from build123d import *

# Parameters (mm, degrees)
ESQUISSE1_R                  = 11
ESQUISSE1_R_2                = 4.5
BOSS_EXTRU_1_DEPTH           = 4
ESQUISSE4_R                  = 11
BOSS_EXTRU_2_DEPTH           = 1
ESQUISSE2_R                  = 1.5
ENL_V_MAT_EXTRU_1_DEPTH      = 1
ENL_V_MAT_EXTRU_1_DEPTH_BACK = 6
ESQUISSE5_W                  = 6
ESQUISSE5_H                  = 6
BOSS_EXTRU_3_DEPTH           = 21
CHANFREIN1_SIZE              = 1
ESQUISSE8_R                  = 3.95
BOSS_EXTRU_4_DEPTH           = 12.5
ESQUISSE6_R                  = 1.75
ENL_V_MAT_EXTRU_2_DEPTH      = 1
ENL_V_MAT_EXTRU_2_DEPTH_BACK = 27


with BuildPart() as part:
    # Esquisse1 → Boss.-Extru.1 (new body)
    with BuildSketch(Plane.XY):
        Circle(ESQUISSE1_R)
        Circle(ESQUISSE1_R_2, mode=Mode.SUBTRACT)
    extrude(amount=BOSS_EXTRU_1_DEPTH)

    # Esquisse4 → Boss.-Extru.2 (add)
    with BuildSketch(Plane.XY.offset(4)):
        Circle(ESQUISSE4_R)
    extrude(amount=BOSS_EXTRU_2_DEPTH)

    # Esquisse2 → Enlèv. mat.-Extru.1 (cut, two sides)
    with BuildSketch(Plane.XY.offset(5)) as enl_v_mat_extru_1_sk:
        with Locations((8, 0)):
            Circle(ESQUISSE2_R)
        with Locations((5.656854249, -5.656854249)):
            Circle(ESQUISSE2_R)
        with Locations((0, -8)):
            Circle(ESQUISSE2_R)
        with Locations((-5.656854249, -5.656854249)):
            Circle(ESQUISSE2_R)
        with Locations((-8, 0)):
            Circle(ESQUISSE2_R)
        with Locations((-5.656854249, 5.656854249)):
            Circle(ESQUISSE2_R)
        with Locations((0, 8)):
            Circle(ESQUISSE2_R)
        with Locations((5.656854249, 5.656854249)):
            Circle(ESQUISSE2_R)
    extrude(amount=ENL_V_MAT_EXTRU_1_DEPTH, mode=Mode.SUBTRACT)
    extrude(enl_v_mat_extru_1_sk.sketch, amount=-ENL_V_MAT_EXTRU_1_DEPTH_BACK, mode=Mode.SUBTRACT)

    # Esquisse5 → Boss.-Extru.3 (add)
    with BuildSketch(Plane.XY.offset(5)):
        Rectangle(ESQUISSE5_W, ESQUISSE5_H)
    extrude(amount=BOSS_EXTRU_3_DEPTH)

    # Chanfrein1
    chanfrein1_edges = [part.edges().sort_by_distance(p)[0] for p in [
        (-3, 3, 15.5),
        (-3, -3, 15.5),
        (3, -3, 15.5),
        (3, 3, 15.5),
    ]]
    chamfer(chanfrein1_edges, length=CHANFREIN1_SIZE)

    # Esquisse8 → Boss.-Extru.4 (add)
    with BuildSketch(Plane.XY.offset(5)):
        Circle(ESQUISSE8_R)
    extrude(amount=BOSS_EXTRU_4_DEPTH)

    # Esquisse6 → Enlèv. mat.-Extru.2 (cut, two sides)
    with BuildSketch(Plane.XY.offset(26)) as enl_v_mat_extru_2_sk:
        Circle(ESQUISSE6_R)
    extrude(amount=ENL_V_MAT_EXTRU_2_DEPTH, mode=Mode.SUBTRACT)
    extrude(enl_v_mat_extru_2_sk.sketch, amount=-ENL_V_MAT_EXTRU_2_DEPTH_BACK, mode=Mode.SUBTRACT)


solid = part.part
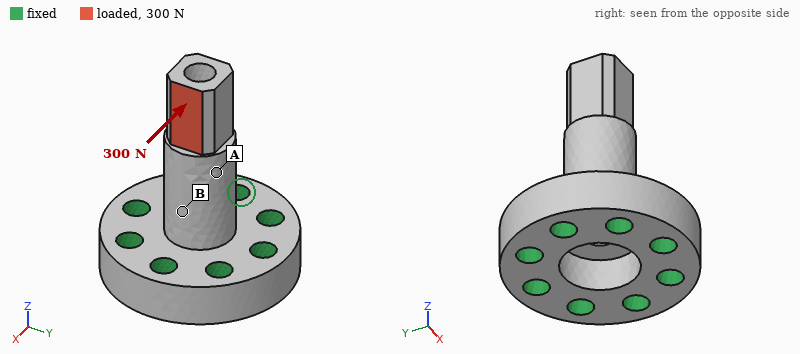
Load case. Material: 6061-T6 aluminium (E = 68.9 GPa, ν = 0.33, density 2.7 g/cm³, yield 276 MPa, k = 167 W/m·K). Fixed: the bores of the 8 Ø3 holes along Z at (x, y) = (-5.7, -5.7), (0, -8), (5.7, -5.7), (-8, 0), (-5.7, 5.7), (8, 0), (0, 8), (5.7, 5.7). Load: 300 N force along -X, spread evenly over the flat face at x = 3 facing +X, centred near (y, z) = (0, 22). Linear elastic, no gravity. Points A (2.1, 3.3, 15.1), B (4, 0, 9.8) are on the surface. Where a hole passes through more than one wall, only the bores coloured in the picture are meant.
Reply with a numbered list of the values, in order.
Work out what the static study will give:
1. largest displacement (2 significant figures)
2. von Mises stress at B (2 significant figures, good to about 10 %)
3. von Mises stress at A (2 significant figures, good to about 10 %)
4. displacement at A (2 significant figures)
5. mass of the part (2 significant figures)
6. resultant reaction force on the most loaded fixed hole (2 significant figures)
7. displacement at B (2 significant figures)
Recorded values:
1. 0.11 mm
2. 76 MPa
3. 26 MPa
4. 0.043 mm
5. 5.5 g
6. 290 N
7. 0.023 mm
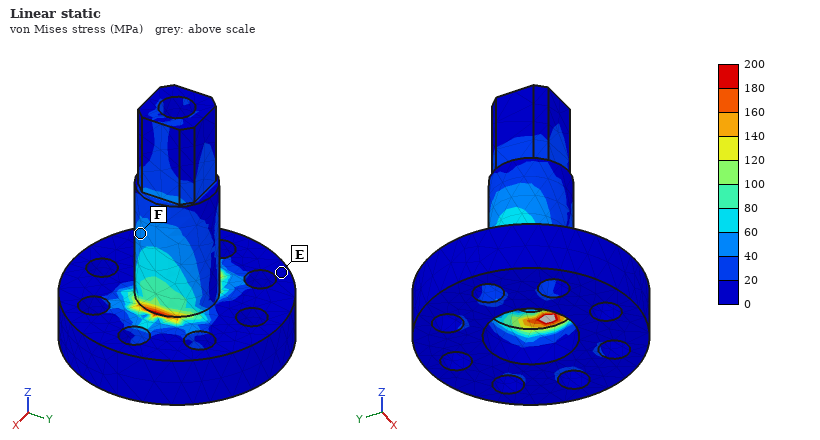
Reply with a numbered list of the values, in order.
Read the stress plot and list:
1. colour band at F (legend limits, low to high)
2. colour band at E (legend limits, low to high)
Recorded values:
1. 40 to 60 MPa
2. 0 to 20 MPa
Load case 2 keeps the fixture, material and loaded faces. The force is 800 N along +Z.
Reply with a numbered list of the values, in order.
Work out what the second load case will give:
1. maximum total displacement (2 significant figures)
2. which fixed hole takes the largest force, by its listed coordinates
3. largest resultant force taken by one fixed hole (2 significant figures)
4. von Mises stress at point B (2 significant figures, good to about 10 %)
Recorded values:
1. 77 µm
2. (8, 0)
3. 250 N
4. 69 MPa
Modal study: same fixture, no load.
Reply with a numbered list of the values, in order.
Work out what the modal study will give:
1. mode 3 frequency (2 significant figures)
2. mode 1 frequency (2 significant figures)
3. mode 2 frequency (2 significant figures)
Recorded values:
1. 41 kHz
2. 11 kHz
3. 11 kHz
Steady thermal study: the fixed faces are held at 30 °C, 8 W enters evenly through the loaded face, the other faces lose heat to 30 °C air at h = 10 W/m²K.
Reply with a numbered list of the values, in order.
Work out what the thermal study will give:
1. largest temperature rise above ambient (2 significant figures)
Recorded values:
1. 31 K
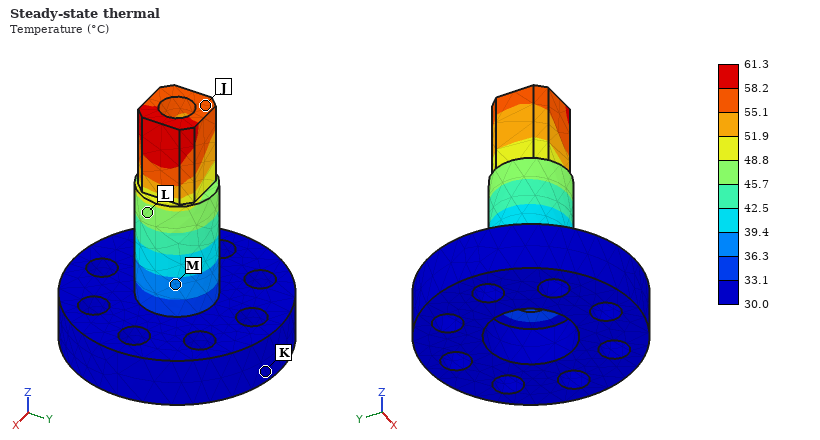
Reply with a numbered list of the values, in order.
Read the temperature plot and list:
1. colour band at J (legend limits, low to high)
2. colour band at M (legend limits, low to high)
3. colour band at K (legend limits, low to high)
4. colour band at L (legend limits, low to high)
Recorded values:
1. 55.1 to 58.2 °C
2. 36.3 to 39.4 °C
3. 30.0 to 33.1 °C
4. 45.7 to 48.8 °C
